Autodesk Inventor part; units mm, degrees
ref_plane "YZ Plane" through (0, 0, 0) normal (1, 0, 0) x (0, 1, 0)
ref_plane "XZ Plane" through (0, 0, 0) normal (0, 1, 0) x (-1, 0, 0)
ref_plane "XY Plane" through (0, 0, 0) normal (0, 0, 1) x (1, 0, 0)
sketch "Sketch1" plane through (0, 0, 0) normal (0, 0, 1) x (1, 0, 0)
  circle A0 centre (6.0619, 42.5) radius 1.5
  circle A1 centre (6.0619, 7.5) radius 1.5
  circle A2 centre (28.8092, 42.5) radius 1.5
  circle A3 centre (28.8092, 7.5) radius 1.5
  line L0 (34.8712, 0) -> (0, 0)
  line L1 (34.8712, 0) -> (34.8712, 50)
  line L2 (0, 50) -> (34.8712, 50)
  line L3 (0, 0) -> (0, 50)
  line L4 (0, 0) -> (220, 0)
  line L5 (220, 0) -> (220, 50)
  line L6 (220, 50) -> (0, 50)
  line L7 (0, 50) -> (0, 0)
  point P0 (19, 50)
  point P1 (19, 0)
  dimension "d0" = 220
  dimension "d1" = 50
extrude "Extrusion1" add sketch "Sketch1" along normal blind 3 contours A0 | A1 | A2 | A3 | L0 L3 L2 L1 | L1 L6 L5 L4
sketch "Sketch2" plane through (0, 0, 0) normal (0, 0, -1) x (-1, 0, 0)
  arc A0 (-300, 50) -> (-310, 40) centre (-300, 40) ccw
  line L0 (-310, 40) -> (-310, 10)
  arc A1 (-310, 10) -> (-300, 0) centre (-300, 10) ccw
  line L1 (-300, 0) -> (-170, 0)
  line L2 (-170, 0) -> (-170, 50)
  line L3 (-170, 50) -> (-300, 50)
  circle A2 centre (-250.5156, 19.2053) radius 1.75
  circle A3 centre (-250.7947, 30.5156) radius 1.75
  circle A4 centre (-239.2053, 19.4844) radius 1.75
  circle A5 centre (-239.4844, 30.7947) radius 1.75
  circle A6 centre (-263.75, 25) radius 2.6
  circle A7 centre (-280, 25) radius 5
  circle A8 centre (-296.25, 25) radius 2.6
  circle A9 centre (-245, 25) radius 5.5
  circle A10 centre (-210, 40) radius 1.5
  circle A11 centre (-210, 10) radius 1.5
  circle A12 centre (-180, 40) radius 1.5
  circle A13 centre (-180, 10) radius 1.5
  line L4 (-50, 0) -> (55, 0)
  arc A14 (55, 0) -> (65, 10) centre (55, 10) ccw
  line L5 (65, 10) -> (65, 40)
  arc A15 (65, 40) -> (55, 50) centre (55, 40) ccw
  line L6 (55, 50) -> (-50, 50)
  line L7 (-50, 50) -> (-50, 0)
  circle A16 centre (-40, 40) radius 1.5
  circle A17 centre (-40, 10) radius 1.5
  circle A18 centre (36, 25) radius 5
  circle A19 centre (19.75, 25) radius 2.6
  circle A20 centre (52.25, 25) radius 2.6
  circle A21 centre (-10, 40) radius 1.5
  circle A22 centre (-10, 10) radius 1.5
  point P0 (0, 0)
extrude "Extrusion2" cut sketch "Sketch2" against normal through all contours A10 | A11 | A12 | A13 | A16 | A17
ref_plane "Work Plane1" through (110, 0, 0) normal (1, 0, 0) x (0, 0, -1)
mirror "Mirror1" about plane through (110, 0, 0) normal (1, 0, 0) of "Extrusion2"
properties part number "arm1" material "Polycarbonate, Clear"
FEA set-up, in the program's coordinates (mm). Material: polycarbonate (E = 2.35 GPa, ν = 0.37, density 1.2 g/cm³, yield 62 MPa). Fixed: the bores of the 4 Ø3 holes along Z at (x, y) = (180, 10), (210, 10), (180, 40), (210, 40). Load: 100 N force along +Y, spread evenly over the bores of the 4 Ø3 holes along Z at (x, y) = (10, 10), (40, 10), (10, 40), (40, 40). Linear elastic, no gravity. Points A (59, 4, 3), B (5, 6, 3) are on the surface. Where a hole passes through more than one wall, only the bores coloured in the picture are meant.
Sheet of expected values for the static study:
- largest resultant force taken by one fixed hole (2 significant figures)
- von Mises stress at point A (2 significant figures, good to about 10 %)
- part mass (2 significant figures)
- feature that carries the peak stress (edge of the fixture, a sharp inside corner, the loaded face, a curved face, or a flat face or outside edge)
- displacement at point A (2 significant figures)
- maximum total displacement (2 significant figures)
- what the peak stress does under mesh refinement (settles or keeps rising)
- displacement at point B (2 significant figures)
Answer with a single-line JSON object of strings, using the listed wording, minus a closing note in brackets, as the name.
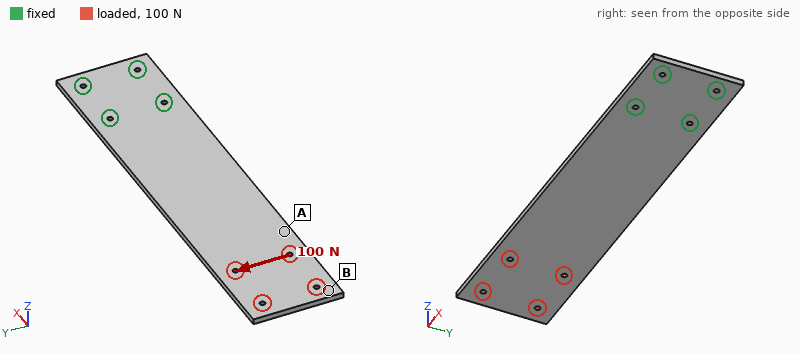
{"largest resultant force taken by one fixed hole": "380 N", "von Mises stress at point A": "2.3 MPa", "part mass": "39 g", "feature that carries the peak stress": "edge of the fixture", "displacement at point A": "1.5 mm", "maximum total displacement": "2.5 mm", "what the peak stress does under mesh refinement": "keeps rising", "displacement at point B": "2.4 mm"}
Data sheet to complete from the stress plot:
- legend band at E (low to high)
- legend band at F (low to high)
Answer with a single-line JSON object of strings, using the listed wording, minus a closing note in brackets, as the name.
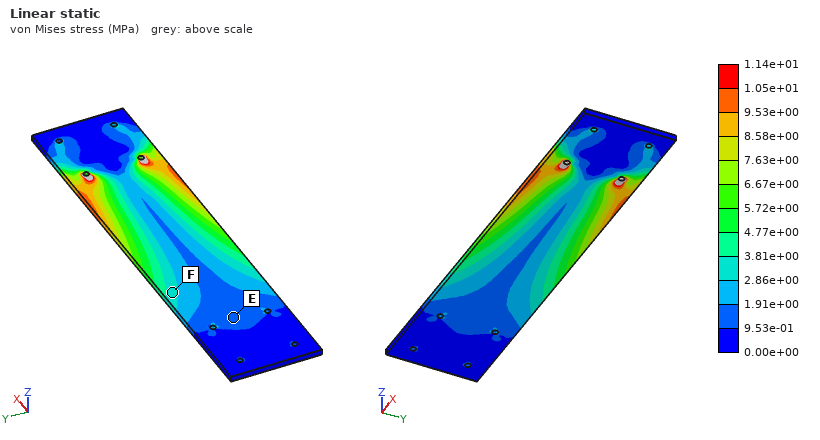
{"legend band at E": "9.53e-01 to 1.91e+00 MPa", "legend band at F": "2.86e+00 to 3.81e+00 MPa"}
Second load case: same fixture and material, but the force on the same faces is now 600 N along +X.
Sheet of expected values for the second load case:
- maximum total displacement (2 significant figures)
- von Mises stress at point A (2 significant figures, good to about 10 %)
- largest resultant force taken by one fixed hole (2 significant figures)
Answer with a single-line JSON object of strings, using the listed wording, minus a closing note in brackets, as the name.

{"maximum total displacement": "0.29 mm", "von Mises stress at point A": "4.0 MPa", "largest resultant force taken by one fixed hole": "240 N"}
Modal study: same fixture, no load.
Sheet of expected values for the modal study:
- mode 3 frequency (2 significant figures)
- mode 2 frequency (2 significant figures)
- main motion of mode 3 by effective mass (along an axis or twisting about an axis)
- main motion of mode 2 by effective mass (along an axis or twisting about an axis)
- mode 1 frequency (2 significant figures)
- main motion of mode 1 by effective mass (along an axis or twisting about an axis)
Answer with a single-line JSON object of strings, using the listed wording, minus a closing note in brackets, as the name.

{"mode 3 frequency": "150 Hz", "mode 2 frequency": "130 Hz", "main motion of mode 3 by effective mass": "twisting about X", "main motion of mode 2 by effective mass": "along Z", "mode 1 frequency": "21 Hz", "main motion of mode 1 by effective mass": "along Z"}
